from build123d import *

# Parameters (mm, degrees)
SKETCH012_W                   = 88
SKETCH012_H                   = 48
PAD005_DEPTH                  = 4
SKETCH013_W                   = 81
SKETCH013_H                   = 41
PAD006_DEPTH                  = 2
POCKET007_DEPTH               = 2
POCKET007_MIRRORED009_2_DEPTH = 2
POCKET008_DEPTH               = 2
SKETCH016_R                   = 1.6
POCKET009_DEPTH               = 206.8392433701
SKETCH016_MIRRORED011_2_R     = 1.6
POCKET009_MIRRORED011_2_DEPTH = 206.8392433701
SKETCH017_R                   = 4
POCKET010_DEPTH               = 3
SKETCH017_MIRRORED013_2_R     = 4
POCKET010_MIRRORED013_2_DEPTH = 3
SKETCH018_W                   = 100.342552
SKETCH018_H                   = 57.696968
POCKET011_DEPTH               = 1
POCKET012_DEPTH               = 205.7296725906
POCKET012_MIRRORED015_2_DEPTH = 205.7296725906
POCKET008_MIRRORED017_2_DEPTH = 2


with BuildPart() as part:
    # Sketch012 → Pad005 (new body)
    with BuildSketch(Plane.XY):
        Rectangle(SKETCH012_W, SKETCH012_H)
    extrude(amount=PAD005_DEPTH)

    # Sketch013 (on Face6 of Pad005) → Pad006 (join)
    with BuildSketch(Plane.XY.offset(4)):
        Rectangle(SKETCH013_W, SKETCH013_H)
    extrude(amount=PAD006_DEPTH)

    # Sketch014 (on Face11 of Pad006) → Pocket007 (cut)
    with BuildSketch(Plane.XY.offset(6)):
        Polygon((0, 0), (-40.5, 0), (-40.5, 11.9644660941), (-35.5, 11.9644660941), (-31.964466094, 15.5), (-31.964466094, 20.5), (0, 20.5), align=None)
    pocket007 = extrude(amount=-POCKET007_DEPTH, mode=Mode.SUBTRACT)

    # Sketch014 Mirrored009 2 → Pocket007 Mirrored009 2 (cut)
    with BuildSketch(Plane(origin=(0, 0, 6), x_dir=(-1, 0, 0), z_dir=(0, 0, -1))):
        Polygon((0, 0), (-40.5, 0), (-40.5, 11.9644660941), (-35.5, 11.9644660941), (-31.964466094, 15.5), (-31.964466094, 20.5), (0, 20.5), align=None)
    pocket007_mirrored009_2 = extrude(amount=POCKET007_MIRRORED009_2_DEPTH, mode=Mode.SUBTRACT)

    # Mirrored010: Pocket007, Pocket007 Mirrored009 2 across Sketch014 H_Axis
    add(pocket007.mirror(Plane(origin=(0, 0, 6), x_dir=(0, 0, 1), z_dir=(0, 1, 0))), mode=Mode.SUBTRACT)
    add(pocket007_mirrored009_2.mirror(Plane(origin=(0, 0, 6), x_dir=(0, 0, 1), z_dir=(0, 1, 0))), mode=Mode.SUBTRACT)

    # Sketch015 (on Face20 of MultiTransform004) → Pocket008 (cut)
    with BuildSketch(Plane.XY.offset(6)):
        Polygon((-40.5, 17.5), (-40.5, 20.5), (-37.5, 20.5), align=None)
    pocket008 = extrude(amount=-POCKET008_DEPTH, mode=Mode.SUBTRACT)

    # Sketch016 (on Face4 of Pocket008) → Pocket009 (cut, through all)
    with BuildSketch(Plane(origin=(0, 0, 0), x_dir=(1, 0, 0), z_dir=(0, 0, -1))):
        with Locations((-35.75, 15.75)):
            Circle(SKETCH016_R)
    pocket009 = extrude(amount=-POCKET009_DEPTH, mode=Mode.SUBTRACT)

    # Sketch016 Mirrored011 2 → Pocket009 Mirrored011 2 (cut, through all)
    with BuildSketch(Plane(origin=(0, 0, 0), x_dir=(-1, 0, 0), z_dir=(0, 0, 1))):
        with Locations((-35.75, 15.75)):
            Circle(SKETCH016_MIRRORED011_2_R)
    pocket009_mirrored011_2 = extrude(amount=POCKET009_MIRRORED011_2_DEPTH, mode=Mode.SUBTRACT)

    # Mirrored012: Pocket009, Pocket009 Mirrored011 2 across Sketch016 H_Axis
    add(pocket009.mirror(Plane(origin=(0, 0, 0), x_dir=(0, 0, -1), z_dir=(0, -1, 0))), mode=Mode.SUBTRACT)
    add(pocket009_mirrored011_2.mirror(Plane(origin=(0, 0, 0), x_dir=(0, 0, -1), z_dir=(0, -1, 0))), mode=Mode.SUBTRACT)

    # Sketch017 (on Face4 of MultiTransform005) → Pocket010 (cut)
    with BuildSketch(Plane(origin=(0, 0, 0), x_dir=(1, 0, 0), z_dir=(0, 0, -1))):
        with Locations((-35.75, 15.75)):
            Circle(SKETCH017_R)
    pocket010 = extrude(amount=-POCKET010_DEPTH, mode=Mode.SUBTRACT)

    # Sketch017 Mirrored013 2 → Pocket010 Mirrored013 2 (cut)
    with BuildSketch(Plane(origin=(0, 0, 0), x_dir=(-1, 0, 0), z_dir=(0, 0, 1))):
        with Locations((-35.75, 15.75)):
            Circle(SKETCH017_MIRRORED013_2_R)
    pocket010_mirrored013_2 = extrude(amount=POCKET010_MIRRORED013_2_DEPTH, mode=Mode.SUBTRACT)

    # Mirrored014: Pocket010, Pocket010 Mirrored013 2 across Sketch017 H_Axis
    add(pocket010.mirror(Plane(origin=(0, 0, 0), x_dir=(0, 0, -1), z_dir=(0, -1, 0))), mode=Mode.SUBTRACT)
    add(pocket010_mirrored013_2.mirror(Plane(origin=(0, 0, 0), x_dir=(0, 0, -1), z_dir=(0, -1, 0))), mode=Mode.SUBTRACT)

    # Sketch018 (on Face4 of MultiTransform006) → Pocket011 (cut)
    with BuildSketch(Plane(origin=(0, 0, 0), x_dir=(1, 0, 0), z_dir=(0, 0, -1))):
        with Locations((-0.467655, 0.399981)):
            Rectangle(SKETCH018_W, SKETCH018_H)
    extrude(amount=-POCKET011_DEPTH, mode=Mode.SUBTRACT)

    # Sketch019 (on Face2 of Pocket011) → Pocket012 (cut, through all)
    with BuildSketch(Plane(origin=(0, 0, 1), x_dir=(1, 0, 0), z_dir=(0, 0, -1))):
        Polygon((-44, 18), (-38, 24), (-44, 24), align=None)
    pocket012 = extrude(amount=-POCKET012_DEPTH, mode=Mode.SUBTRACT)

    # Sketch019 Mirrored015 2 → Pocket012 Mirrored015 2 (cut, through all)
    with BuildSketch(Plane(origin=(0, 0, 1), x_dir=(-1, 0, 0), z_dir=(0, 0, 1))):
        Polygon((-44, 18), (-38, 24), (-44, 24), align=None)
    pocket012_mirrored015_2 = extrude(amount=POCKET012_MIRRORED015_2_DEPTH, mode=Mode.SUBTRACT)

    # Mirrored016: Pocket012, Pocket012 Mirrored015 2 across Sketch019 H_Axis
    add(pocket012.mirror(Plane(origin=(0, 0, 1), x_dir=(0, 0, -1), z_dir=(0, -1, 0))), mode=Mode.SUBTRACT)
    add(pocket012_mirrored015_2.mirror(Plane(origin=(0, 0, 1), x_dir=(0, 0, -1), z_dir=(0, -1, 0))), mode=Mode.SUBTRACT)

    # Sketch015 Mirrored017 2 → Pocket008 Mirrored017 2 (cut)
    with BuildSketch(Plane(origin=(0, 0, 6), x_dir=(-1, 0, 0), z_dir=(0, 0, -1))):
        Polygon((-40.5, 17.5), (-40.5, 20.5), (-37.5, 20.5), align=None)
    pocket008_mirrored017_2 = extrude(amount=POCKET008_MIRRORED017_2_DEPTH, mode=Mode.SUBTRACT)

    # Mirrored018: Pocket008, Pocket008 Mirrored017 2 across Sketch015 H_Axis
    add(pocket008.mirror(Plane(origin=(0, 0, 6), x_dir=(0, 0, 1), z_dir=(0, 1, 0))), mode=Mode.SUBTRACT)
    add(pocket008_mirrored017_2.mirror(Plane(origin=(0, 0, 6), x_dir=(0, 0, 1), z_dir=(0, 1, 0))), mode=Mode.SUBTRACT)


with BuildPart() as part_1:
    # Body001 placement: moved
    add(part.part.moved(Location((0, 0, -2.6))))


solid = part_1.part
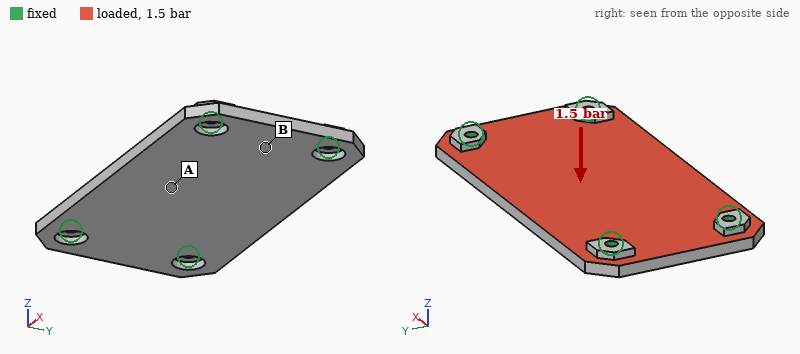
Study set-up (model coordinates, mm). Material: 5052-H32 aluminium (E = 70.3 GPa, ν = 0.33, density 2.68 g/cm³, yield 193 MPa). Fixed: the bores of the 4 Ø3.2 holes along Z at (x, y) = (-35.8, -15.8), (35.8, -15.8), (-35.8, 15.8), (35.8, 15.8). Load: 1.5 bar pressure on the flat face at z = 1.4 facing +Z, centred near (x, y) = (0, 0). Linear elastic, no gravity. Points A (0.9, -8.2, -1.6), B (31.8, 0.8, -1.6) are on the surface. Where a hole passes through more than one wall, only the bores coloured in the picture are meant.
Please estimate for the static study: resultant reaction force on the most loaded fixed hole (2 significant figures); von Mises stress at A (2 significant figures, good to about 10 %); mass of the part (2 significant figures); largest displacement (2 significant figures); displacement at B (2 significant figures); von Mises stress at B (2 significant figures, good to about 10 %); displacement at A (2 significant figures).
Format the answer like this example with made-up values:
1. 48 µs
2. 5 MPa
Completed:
1. 290 N
2. 24 MPa
3. 33 g
4. 81 µm
5. 14 µm
6. 15 MPa
7. 78 µm
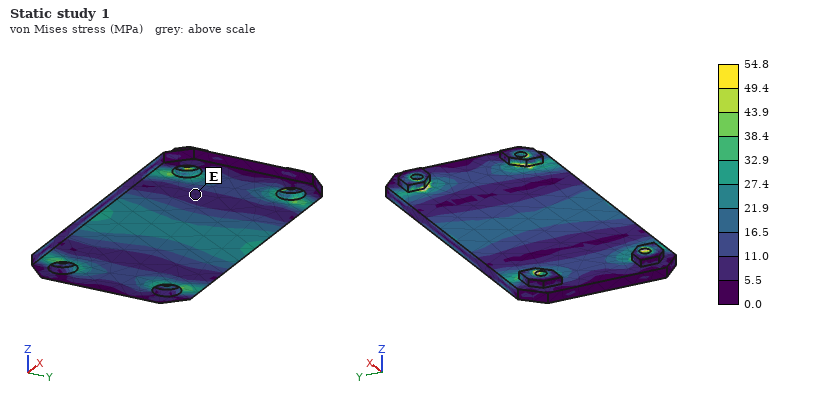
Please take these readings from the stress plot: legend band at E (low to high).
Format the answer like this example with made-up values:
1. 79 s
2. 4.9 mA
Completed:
1. 5.5 to 11.0 MPa
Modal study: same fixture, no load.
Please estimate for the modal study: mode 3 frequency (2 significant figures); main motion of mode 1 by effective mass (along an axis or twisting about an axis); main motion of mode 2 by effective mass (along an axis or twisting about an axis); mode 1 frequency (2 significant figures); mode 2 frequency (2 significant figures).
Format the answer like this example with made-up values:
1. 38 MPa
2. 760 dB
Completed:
1. 7200 Hz
2. along Z
3. twisting about X
4. 2800 Hz
5. 4200 Hz
